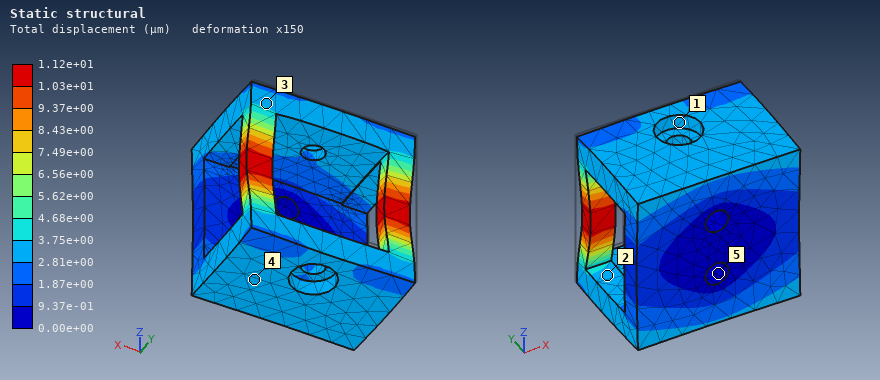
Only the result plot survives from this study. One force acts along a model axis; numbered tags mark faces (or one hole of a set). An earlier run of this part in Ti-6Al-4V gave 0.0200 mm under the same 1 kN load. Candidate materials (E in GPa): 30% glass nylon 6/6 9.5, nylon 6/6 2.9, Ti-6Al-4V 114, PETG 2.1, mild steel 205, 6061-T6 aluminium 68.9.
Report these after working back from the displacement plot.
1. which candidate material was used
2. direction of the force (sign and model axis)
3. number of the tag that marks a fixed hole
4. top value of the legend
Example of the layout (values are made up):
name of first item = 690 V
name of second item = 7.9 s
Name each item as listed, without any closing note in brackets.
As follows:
which candidate material was used = mild steel
direction of the force = -Y
number of the tag that marks a fixed hole = 5
top value of the legend = 1.12e+01 µm
